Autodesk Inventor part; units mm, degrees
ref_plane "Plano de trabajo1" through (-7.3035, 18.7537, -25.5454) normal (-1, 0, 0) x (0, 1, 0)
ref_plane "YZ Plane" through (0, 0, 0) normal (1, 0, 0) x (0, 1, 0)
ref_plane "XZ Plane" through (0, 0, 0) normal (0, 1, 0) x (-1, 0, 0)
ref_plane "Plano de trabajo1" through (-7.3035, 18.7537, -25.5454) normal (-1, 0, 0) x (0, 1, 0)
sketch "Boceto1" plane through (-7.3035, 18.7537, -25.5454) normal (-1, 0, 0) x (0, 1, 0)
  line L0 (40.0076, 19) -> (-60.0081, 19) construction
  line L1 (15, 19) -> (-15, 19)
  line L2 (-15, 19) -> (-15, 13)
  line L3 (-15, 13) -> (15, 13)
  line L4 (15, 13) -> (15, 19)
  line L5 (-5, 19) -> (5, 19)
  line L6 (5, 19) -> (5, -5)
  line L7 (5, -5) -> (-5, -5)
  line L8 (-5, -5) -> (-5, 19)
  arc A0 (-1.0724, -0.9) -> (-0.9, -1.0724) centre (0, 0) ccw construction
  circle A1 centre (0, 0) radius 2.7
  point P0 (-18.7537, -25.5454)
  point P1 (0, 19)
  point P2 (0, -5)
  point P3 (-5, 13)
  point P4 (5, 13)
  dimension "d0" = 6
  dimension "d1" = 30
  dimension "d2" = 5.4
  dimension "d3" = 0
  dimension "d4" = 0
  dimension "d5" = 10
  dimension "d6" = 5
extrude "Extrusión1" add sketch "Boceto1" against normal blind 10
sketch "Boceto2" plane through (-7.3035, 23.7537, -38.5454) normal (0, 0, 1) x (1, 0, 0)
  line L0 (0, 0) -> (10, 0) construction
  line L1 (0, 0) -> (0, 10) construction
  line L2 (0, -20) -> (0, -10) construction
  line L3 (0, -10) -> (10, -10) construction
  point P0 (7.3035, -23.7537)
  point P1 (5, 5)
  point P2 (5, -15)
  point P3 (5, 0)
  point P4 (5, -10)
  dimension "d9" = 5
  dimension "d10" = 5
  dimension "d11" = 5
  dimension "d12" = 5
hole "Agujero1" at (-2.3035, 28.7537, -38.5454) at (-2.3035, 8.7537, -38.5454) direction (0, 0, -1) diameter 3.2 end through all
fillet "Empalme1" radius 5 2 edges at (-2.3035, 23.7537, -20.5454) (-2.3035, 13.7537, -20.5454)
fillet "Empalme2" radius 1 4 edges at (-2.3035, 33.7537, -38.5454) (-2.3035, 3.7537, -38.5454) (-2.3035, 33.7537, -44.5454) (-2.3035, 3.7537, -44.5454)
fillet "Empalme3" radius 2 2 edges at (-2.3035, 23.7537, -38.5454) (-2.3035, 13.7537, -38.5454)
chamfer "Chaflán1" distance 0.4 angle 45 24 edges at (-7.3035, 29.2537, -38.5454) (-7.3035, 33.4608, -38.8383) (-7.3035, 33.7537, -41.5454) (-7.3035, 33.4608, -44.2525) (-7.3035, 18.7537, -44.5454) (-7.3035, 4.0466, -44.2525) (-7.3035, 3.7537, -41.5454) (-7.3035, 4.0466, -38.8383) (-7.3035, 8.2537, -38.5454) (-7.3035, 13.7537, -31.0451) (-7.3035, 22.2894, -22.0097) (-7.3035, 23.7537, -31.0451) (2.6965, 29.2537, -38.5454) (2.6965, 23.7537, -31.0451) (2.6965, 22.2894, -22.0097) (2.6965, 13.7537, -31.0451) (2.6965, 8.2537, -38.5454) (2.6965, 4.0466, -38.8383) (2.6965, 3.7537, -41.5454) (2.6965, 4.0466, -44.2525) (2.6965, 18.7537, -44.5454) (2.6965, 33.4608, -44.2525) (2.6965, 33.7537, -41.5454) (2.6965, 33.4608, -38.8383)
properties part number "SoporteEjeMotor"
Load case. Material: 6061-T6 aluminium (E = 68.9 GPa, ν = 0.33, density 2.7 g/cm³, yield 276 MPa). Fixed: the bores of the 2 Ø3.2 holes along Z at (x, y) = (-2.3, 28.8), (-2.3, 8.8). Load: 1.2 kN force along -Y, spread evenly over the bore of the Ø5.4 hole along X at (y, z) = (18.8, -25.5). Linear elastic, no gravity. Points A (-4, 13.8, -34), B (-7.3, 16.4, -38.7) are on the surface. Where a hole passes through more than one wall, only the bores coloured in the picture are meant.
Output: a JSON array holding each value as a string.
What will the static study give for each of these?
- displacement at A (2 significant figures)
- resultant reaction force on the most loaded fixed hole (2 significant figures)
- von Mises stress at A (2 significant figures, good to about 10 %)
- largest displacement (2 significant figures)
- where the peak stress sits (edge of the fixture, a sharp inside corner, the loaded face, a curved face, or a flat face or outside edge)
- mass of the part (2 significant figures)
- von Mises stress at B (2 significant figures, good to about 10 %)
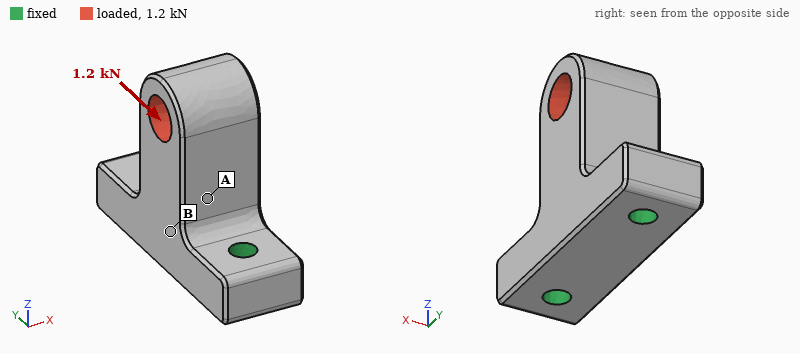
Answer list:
["15 µm", "1.3 kN", "64 MPa", "57 µm", "a curved face", "8.5 g", "19 MPa"]
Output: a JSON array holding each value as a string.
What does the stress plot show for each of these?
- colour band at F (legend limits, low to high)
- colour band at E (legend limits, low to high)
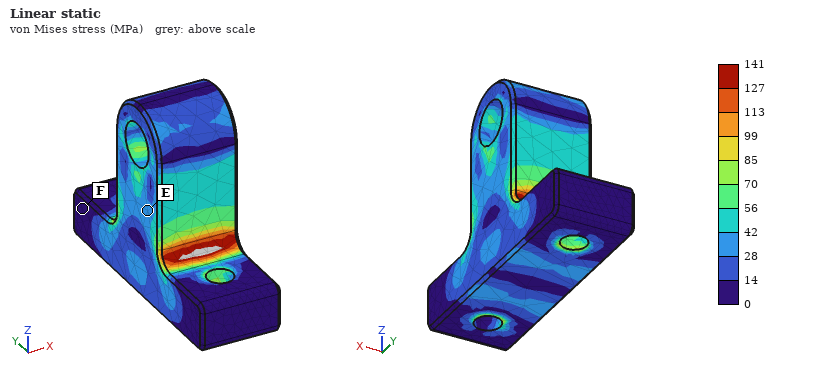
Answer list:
["0 to 14 MPa", "28 to 42 MPa"]
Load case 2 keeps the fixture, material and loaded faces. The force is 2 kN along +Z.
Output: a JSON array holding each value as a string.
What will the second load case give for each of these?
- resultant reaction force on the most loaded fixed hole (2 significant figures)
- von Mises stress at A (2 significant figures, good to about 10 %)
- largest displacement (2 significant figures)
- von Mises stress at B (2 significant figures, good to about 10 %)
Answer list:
["1.1 kN", "25 MPa", "14 µm", "12 MPa"]
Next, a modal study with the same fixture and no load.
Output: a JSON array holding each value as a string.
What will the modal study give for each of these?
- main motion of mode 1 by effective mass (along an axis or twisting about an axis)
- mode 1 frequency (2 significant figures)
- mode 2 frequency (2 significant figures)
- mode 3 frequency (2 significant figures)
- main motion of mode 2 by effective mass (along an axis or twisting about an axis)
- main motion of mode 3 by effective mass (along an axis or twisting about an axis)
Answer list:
["along X", "12 kHz", "20 kHz", "36 kHz", "along Y", "along Z"]
